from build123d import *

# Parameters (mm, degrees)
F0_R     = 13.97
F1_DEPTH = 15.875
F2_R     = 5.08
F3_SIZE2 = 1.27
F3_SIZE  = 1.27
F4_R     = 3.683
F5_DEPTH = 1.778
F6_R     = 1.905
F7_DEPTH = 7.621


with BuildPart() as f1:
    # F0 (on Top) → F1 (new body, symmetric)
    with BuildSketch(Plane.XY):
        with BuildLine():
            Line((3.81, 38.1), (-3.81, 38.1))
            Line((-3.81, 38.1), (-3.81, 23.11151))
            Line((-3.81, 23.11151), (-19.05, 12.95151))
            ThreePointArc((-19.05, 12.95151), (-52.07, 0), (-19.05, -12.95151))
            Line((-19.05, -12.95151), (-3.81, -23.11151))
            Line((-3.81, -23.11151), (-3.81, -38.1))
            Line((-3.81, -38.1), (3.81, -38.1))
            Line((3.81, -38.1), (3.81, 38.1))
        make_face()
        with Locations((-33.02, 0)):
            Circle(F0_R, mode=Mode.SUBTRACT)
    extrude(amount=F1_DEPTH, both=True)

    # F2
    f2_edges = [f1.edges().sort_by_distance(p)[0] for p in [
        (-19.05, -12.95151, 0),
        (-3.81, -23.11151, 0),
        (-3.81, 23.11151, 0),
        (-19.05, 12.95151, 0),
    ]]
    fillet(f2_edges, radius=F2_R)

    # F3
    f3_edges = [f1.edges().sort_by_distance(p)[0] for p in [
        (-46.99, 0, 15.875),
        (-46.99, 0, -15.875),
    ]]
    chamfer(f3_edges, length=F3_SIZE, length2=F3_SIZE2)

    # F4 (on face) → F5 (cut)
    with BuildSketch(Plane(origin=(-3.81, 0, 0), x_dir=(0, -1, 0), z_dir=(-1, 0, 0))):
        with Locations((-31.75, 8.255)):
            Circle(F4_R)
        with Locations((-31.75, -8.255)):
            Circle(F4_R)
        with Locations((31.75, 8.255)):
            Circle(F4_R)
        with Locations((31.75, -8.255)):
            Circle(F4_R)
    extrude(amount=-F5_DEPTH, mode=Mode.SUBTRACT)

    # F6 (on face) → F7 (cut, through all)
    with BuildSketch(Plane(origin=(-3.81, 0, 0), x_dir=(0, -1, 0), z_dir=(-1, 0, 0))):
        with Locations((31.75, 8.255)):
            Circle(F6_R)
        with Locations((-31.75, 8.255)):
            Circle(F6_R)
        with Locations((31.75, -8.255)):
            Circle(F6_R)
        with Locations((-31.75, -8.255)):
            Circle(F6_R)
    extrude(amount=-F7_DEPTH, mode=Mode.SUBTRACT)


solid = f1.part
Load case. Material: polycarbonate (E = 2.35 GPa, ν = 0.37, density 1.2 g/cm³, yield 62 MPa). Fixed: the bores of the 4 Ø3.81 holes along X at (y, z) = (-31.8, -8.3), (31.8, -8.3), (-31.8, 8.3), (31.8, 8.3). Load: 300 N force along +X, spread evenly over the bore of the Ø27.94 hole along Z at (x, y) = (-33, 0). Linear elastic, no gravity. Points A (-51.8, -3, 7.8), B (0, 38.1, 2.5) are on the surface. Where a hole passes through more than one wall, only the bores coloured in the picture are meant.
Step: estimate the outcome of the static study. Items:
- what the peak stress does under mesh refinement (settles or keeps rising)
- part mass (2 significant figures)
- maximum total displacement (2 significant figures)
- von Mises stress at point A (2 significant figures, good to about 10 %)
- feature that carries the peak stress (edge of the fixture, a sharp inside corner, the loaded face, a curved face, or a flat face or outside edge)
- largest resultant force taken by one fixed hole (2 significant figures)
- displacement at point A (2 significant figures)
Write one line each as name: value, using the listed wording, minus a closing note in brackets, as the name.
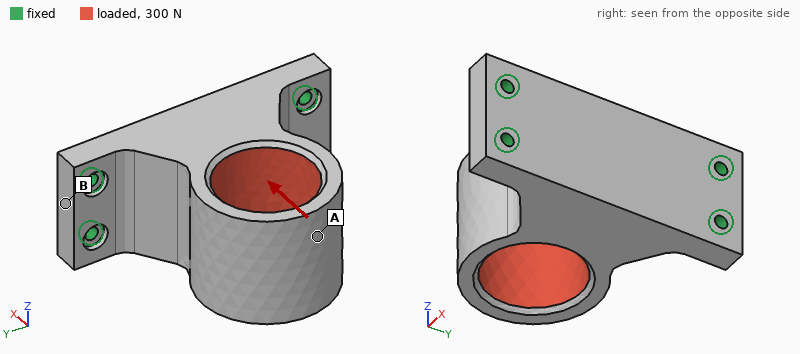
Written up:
what the peak stress does under mesh refinement: keeps rising
part mass: 59 g
maximum total displacement: 63 µm
von Mises stress at point A: 1.1 MPa
feature that carries the peak stress: edge of the fixture
largest resultant force taken by one fixed hole: 97 N
displacement at point A: 60 µm
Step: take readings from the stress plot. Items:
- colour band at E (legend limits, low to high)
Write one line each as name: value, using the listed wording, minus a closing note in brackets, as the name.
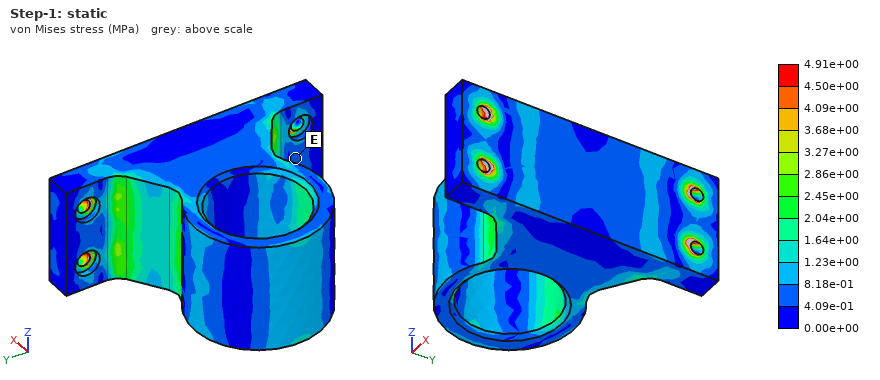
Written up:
colour band at E: 4.09e-01 to 8.18e-01 MPa
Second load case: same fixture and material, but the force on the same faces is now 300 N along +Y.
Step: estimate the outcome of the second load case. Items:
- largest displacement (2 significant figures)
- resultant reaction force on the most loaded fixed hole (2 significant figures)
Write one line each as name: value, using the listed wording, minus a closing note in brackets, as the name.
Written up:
largest displacement: 0.29 mm
resultant reaction force on the most loaded fixed hole: 120 N
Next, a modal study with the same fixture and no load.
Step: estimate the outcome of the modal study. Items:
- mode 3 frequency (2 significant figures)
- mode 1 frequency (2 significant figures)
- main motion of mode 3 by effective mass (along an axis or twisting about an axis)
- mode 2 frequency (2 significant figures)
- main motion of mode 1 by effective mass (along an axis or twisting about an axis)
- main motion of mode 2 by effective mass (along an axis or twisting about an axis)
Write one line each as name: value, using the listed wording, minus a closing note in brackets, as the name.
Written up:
mode 3 frequency: 2200 Hz
mode 1 frequency: 910 Hz
main motion of mode 3 by effective mass: along X
mode 2 frequency: 1300 Hz
main motion of mode 1 by effective mass: along Z
main motion of mode 2 by effective mass: along Y
